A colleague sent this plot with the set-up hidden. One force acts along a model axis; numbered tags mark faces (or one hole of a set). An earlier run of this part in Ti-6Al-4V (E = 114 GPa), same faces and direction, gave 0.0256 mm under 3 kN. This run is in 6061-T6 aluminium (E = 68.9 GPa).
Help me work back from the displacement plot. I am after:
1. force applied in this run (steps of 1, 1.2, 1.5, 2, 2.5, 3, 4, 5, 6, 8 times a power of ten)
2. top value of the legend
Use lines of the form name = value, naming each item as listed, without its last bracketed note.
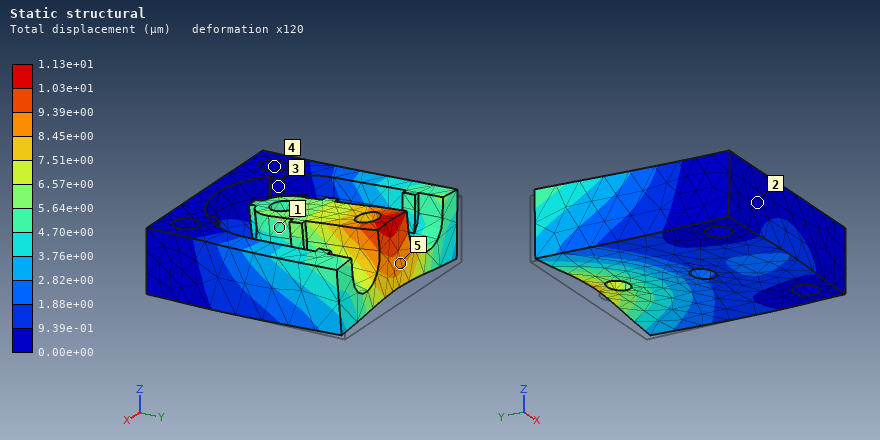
force applied in this run = 800 N
top value of the legend = 1.13e+01 µm
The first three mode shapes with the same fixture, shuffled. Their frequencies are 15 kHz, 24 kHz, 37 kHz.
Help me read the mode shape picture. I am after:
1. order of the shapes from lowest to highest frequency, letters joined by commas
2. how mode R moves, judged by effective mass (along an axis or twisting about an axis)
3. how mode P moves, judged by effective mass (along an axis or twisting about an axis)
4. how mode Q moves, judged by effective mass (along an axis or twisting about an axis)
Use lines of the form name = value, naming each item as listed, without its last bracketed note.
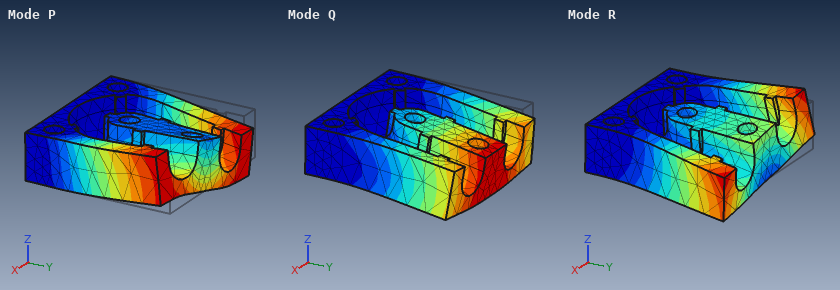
order of the shapes from lowest to highest frequency, letters joined by commas = Q, R, P
how mode R moves, judged by effective mass = along X
how mode P moves, judged by effective mass = along X
how mode Q moves, judged by effective mass = along Z
